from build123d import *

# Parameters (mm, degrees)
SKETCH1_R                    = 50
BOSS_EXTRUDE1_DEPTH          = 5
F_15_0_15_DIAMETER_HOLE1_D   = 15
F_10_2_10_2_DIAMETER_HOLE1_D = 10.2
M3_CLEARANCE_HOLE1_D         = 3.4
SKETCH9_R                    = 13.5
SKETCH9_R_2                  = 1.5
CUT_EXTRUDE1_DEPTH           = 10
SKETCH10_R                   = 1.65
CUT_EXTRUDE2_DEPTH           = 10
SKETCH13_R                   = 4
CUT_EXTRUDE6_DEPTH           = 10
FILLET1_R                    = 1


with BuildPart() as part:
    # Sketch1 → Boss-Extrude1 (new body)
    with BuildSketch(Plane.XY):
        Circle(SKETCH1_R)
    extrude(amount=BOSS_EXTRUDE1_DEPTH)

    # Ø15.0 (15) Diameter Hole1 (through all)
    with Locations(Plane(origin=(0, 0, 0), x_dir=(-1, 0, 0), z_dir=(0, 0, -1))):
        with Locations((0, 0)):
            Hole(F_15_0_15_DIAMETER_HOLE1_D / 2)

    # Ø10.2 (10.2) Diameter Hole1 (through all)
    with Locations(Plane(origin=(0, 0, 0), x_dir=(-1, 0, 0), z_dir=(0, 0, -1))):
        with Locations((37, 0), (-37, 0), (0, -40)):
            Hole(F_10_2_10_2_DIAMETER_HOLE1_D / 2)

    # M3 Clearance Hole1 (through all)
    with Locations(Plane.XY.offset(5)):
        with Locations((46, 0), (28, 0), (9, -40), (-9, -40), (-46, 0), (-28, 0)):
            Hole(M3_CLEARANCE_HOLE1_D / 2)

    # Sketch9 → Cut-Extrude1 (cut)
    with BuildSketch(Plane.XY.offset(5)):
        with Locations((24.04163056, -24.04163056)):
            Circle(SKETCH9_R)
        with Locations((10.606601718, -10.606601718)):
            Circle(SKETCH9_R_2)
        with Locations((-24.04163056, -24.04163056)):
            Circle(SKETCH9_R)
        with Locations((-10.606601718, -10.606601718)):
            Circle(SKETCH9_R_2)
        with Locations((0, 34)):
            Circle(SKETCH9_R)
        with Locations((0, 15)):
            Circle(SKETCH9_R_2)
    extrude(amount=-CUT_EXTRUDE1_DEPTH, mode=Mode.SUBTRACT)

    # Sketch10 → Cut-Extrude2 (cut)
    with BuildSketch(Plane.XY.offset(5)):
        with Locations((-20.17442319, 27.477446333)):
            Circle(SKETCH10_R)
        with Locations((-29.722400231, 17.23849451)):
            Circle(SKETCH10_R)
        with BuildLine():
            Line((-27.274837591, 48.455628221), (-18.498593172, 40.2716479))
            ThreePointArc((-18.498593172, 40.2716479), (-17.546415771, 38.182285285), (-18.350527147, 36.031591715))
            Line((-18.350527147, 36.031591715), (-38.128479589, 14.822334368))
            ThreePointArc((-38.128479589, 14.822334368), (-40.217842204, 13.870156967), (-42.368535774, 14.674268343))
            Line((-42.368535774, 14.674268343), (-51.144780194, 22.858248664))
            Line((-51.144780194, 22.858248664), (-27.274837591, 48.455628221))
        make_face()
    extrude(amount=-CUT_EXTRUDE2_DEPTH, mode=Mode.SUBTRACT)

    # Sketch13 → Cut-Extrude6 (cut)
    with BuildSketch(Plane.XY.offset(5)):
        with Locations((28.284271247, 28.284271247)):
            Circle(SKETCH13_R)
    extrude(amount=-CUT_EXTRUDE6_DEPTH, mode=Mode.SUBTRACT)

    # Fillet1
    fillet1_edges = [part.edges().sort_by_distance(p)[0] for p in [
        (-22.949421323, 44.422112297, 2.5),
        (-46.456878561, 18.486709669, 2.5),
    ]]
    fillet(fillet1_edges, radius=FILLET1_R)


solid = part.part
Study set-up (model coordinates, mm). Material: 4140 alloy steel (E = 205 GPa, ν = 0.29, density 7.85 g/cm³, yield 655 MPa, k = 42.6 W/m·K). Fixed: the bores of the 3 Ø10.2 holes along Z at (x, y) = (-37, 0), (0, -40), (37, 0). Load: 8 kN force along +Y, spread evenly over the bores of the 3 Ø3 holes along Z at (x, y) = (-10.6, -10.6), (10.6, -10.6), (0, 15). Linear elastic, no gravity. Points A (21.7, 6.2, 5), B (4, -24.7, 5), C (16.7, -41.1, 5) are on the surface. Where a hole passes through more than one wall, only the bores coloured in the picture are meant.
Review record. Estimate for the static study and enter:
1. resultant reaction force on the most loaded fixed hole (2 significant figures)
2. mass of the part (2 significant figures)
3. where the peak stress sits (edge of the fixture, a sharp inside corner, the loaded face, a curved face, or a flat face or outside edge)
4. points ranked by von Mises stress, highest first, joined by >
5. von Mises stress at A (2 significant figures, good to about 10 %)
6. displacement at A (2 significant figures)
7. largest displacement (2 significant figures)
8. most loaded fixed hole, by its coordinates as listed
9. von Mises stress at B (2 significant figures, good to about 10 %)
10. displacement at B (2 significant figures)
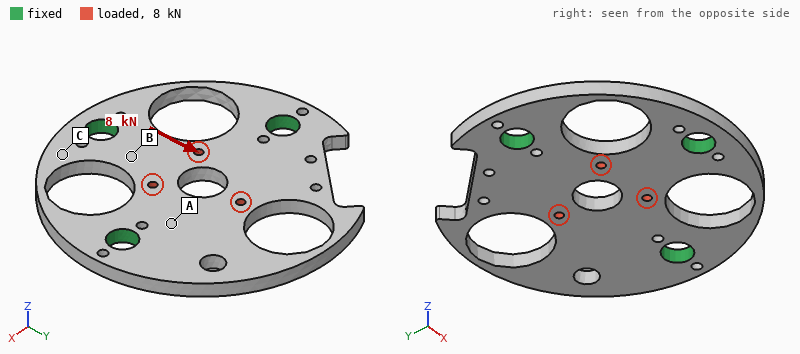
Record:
4.2 kN
200 g
the loaded face
B > A > C
22 MPa
3.7 µm
11 µm
(0, -40)
36 MPa
2.5 µm
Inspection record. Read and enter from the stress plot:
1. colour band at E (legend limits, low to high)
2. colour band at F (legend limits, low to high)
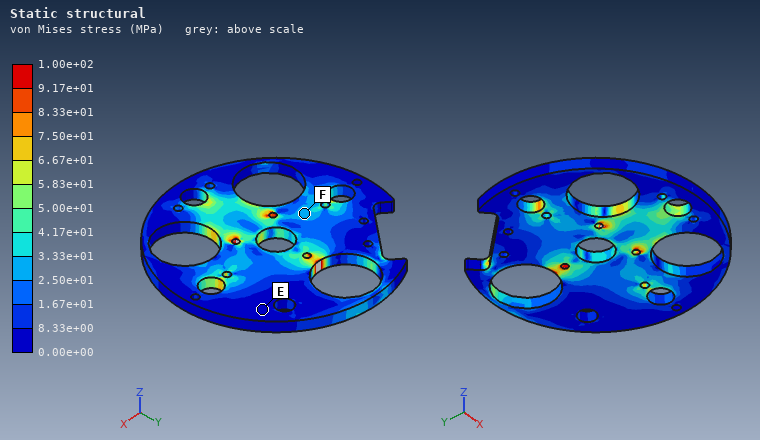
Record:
0.00e+00 to 8.33e+00 MPa
2.50e+01 to 3.33e+01 MPa
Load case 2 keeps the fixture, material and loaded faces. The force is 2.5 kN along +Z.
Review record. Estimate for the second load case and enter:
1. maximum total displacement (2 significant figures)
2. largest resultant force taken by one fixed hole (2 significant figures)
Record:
67 µm
940 N
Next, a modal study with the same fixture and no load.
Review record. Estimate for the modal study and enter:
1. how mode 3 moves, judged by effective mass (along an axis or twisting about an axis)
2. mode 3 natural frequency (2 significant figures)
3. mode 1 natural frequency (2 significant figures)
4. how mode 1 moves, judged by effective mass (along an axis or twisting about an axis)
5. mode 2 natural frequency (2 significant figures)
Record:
along Z
6000 Hz
2300 Hz
along Z
4700 Hz
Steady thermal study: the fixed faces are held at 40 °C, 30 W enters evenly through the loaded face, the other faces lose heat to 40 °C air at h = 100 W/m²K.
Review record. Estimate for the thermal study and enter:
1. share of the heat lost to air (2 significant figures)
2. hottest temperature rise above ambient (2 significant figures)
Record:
45 %
39 K
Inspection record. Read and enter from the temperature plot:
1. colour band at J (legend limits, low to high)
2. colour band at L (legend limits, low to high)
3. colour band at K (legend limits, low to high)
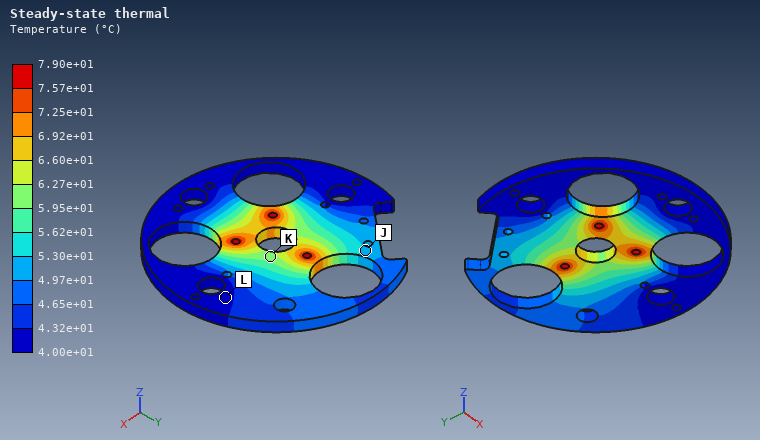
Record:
4.97e+01 to 5.30e+01 °C
4.00e+01 to 4.32e+01 °C
5.95e+01 to 6.27e+01 °C
